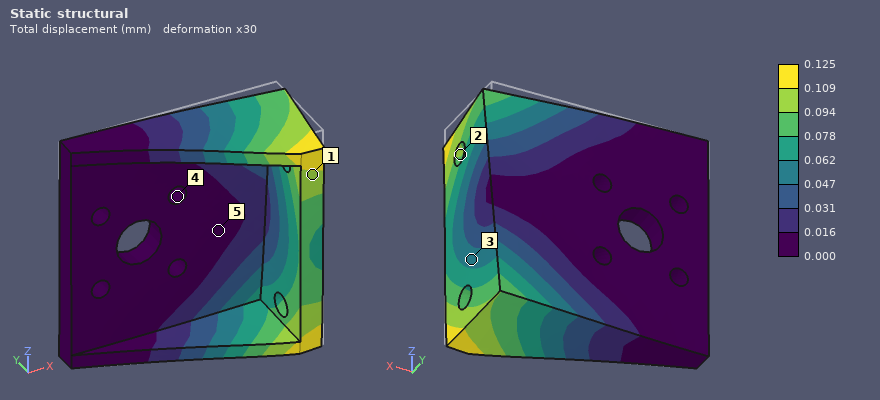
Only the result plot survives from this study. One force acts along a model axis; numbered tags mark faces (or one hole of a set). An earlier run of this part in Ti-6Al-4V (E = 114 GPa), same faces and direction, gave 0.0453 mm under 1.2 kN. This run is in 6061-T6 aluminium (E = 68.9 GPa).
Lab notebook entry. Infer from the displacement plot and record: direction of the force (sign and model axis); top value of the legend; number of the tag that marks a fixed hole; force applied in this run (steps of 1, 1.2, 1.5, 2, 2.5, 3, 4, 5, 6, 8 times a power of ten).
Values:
-Z
0.125 mm
4
2 kN
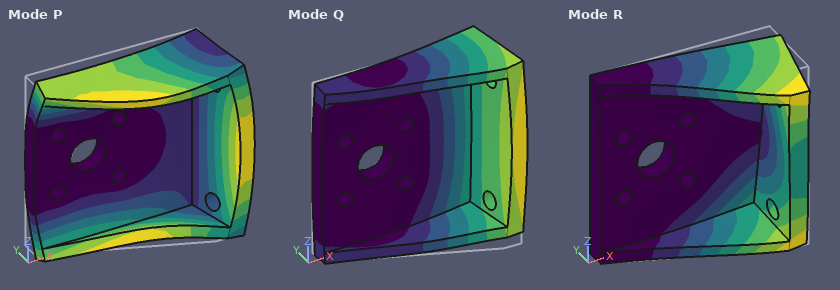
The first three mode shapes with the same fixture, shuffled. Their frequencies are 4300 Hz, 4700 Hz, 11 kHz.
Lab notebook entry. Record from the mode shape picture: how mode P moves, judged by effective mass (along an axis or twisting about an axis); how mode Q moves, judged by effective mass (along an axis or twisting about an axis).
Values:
along Y
along Y
